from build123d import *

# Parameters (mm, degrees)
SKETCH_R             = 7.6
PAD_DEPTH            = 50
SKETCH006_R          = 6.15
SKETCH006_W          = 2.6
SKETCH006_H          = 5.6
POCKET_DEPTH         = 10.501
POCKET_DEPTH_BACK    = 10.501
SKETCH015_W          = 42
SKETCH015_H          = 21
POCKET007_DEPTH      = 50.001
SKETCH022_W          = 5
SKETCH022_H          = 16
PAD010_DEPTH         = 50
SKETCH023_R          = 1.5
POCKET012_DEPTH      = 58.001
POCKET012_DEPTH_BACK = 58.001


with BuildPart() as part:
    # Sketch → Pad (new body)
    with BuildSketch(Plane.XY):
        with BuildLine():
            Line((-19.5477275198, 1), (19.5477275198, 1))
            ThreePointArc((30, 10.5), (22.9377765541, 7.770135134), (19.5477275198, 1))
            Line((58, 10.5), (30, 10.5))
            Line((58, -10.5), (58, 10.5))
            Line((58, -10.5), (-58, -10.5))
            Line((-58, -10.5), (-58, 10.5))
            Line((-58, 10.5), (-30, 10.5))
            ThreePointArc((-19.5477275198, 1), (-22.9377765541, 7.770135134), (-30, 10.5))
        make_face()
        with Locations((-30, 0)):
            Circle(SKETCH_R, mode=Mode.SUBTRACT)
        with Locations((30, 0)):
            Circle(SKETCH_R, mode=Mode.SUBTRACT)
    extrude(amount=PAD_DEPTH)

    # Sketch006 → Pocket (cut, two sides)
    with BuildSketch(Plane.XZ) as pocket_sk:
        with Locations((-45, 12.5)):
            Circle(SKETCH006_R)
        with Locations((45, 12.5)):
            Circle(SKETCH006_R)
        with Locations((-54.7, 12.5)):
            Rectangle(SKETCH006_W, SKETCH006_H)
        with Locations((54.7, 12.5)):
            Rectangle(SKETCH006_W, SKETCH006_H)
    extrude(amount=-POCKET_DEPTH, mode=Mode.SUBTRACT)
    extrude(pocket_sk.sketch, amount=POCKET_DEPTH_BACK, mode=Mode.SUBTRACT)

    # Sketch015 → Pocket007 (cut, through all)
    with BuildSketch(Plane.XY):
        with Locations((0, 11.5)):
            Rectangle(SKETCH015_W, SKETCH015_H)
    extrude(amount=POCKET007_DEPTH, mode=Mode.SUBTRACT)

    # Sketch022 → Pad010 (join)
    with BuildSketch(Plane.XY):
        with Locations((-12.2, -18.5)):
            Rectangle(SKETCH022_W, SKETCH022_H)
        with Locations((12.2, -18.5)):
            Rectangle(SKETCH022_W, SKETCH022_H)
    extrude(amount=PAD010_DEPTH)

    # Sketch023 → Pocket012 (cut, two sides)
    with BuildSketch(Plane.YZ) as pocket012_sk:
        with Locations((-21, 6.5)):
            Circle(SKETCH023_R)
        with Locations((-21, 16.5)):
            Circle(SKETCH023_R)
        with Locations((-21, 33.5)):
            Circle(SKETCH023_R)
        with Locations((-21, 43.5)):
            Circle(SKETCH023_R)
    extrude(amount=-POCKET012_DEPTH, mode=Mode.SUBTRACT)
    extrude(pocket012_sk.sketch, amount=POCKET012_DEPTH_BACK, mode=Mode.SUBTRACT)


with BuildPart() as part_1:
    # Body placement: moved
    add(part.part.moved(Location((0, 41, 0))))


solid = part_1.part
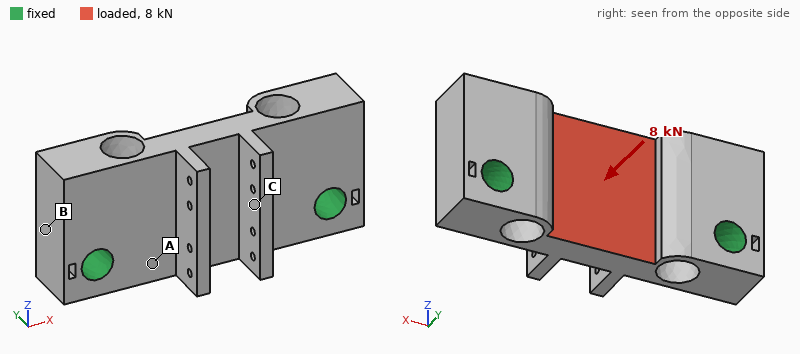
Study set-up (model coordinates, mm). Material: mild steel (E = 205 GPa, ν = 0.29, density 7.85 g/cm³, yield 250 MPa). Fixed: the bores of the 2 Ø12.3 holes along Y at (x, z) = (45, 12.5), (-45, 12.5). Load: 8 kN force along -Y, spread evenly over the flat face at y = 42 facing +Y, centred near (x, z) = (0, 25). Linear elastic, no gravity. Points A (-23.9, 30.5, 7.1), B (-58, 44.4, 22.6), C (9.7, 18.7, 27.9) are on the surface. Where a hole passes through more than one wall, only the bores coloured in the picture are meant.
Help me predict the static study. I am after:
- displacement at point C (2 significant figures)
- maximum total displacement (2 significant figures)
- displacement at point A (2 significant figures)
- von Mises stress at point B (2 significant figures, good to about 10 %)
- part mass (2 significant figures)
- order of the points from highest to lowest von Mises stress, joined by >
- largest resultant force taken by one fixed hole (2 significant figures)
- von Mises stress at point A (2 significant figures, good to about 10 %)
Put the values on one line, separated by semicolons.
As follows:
25 µm; 30 µm; 16 µm; 19 MPa; 660 g; A > B > C; 4.1 kN; 38 MPa
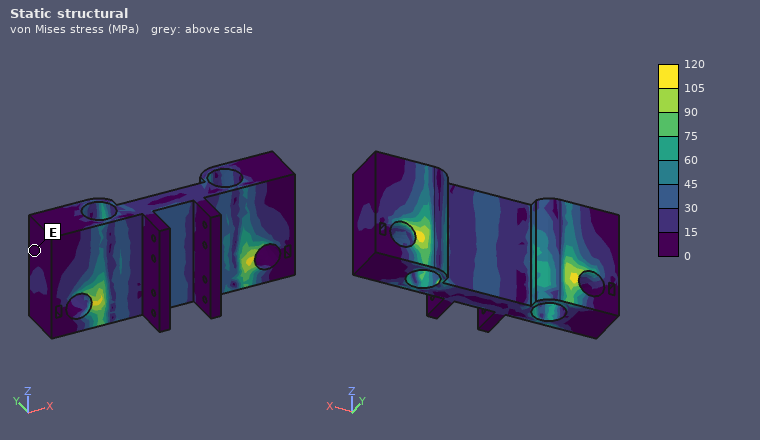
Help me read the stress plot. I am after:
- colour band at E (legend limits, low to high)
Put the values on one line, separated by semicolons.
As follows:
0 to 15 MPa
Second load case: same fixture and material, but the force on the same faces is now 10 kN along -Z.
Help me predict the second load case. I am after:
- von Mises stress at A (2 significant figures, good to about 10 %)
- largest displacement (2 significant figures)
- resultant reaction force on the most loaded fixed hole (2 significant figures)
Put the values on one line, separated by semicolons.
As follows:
13 MPa; 12 µm; 5.2 kN
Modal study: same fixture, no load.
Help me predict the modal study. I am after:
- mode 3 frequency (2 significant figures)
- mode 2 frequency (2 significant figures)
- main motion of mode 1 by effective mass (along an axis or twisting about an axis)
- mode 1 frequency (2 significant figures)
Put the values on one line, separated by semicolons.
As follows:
9100 Hz; 7400 Hz; along Y; 5300 Hz
